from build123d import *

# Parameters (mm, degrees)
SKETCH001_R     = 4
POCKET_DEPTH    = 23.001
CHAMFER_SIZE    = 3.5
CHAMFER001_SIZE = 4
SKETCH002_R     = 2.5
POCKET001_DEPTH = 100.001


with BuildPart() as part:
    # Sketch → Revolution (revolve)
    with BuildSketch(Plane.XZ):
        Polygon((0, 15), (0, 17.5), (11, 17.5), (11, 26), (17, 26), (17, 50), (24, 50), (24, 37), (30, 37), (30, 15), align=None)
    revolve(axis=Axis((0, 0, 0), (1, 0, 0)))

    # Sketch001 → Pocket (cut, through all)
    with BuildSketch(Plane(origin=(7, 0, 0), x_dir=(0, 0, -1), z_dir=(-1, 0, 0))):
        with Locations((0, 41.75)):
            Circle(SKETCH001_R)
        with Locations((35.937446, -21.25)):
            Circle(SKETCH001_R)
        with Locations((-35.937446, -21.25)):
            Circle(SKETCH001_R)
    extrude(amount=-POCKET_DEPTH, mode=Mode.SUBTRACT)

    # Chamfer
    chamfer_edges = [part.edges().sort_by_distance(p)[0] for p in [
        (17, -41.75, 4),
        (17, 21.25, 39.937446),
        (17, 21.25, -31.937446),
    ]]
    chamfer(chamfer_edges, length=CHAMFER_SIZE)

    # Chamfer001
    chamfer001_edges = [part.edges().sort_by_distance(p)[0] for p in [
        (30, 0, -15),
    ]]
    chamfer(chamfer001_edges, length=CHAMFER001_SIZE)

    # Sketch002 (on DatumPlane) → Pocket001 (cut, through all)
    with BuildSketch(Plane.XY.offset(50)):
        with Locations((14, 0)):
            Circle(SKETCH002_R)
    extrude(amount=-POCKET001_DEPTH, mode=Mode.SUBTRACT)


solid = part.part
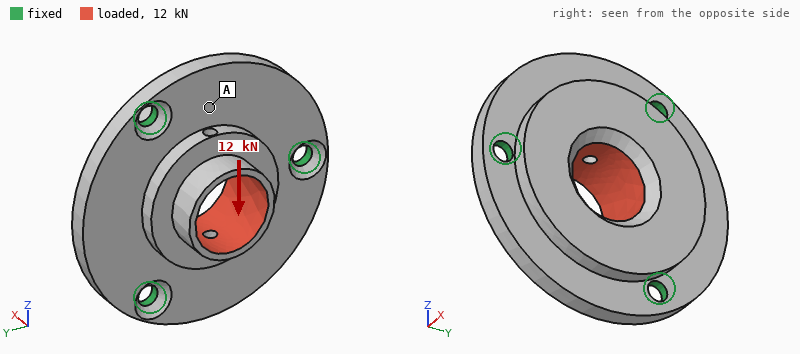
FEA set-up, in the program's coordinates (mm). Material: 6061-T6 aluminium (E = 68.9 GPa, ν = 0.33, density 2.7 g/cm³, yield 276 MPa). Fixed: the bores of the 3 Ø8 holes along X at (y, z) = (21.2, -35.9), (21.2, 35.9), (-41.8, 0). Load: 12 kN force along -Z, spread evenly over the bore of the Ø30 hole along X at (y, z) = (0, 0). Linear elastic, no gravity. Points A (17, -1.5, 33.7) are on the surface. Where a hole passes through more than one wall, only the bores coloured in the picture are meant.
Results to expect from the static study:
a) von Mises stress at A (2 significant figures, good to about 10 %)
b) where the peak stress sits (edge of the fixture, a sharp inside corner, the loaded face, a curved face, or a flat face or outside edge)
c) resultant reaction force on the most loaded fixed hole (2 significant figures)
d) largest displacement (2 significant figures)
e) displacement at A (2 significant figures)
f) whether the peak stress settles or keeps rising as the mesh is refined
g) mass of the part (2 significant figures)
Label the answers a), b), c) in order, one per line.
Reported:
a) 16 MPa
b) edge of the fixture
c) 4.3 kN
d) 54 µm
e) 23 µm
f) keeps rising
g) 220 g
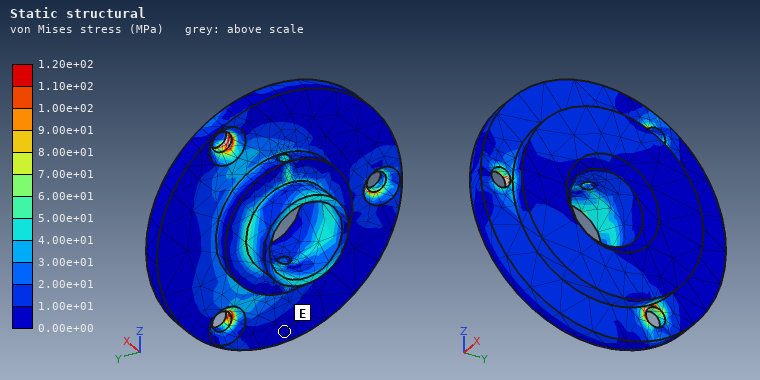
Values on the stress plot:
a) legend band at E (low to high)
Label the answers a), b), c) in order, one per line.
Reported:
a) 0.00e+00 to 1.00e+01 MPa
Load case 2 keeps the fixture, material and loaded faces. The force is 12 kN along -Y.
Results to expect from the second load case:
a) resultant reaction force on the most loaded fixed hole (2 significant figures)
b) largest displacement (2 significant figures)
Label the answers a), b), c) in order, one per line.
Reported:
a) 4.4 kN
b) 57 µm
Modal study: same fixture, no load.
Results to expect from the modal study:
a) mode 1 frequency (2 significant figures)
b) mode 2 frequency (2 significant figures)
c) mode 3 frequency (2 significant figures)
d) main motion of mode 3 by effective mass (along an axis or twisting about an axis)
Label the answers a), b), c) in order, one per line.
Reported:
a) 5400 Hz
b) 5500 Hz
c) 6300 Hz
d) along X
